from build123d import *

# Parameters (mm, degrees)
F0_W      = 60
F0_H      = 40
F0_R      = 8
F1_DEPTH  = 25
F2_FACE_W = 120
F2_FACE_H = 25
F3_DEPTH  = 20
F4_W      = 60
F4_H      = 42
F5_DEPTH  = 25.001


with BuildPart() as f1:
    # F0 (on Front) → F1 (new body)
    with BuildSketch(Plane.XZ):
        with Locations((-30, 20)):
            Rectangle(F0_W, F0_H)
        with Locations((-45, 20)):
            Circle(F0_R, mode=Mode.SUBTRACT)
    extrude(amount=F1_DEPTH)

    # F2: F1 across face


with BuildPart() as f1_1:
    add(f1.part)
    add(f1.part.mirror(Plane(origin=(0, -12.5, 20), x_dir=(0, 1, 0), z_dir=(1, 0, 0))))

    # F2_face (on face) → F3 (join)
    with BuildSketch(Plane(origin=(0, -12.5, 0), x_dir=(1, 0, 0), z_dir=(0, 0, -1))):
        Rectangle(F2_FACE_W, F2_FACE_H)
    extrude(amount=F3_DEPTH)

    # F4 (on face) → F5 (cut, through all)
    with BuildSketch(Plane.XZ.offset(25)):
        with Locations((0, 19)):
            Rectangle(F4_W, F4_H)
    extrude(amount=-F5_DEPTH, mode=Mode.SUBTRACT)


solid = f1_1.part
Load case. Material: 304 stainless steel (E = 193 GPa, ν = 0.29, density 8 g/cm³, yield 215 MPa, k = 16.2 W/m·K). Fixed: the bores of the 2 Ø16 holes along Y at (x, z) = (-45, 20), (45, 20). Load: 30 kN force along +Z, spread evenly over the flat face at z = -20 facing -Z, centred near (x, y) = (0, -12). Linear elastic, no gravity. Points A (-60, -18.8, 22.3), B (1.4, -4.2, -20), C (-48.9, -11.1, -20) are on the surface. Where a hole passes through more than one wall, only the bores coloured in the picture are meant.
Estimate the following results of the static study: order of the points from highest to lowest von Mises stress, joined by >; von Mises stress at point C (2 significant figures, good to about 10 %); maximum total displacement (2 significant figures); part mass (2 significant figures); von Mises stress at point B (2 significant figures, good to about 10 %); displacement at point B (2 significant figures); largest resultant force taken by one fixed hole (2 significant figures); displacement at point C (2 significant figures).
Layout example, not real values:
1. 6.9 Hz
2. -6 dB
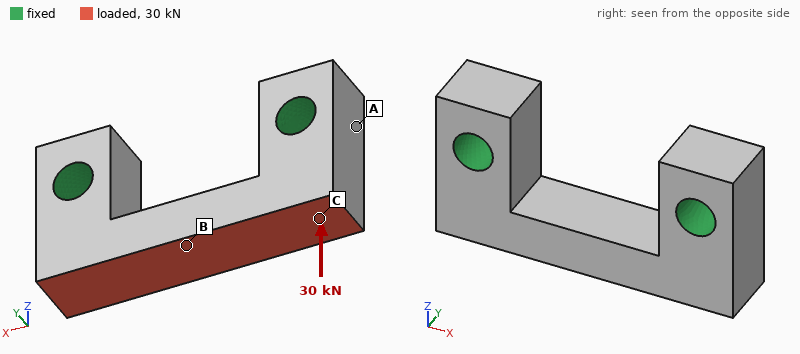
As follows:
1. B > C > A
2. 16 MPa
3. 19 µm
4. 860 g
5. 55 MPa
6. 18 µm
7. 16 kN
8. 3.2 µm
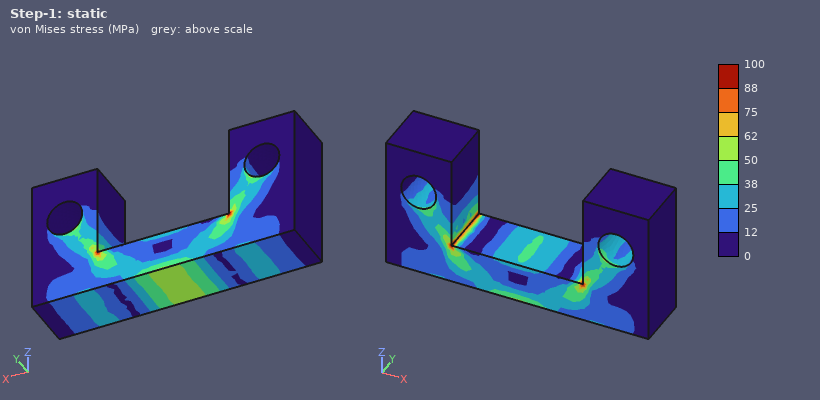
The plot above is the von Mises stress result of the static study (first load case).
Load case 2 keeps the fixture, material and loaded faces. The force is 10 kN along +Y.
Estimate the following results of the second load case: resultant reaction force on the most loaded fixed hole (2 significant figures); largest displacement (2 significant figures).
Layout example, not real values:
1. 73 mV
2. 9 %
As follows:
1. 5.0 kN
2. 22 µm
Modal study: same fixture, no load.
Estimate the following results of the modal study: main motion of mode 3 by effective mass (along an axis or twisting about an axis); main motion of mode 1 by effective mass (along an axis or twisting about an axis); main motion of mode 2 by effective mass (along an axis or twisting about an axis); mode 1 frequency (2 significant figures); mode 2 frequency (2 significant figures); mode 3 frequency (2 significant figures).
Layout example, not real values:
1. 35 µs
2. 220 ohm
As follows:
1. along Z
2. along Y
3. along X
4. 7400 Hz
5. 9900 Hz
6. 11 kHz
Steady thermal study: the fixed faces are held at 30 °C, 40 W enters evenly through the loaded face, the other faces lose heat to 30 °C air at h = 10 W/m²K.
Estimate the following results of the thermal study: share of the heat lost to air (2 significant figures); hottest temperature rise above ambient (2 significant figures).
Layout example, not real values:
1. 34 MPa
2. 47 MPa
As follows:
1. 9.1 %
2. 69 K
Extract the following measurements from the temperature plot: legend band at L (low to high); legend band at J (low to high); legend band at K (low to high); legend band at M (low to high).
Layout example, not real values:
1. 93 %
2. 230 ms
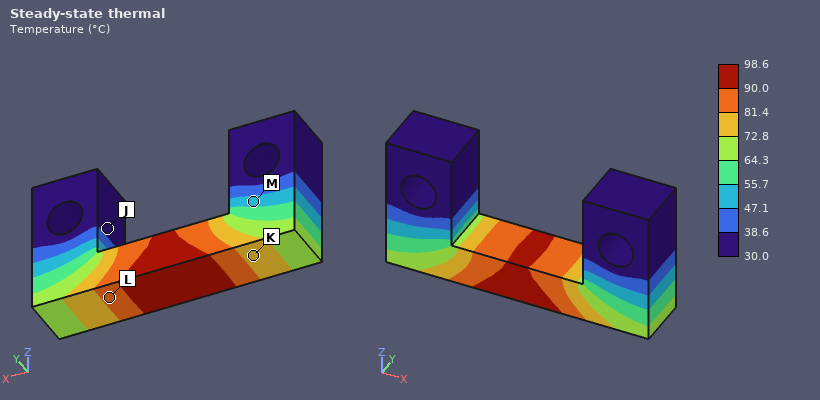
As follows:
1. 81.4 to 90.0 °C
2. 30.0 to 38.6 °C
3. 72.8 to 81.4 °C
4. 47.1 to 55.7 °C
